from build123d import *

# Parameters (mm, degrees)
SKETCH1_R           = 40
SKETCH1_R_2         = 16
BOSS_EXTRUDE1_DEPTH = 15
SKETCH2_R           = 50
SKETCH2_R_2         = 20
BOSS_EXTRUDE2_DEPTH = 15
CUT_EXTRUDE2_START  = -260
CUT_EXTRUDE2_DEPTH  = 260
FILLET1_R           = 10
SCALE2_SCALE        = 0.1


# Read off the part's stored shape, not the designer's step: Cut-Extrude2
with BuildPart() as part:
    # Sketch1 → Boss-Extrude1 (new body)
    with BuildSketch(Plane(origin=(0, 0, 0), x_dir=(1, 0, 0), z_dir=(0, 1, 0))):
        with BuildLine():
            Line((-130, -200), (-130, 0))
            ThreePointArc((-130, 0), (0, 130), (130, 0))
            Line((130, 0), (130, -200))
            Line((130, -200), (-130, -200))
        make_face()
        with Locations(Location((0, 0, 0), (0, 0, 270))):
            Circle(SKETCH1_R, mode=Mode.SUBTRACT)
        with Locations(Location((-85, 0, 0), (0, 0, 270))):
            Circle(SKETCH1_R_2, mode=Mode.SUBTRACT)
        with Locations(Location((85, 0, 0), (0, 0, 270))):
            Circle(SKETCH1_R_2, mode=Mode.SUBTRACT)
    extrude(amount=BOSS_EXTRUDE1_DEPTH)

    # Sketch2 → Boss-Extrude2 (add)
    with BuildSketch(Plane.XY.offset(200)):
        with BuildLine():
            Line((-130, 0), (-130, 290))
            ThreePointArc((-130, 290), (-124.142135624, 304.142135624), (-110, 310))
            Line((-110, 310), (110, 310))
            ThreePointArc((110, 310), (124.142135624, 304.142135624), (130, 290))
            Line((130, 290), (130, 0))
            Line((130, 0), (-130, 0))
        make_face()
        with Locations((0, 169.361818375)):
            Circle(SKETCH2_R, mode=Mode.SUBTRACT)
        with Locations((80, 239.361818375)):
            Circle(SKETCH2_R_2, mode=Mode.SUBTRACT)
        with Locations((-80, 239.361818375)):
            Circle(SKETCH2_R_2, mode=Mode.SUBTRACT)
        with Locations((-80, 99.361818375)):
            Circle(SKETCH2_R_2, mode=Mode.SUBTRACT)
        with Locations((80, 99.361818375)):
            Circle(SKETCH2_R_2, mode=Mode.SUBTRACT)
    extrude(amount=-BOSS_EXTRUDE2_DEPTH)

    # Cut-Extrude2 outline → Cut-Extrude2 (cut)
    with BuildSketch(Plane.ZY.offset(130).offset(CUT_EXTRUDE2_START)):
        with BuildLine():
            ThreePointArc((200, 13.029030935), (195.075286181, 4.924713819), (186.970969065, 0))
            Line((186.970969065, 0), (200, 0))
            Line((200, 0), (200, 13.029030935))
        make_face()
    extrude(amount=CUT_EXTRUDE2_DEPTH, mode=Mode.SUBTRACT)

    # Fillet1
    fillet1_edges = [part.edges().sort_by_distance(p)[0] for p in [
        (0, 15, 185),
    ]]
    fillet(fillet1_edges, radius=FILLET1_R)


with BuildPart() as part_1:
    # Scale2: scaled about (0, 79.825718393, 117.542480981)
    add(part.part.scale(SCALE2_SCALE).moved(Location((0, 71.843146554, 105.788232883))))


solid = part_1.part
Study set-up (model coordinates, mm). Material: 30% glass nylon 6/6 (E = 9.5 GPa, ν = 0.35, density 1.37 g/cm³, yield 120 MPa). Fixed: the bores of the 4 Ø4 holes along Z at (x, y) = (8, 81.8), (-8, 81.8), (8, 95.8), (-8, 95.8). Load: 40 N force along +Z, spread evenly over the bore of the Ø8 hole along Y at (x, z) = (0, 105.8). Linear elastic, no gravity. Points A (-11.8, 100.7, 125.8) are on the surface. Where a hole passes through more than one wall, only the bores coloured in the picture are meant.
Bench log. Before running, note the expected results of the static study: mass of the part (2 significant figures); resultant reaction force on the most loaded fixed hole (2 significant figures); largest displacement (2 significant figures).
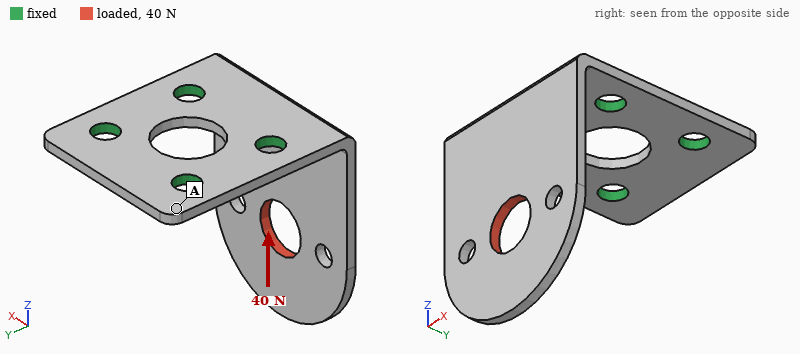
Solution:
2.8 g
20 N
0.57 mm
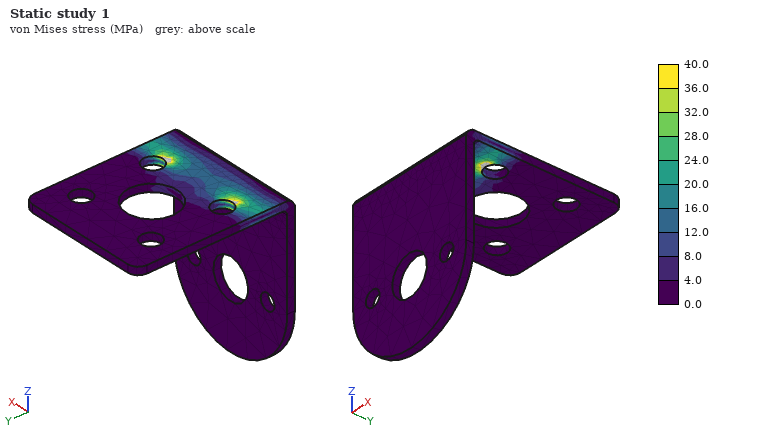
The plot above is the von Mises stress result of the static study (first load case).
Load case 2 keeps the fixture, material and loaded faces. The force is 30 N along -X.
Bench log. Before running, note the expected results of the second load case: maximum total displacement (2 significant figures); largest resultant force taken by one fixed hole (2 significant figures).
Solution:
0.34 mm
38 N
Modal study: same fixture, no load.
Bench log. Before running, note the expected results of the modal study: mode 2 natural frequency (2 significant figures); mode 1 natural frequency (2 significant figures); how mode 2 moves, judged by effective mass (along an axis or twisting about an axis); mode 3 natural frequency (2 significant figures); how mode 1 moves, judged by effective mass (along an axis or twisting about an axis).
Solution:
1500 Hz
560 Hz
along X
2300 Hz
along Y
